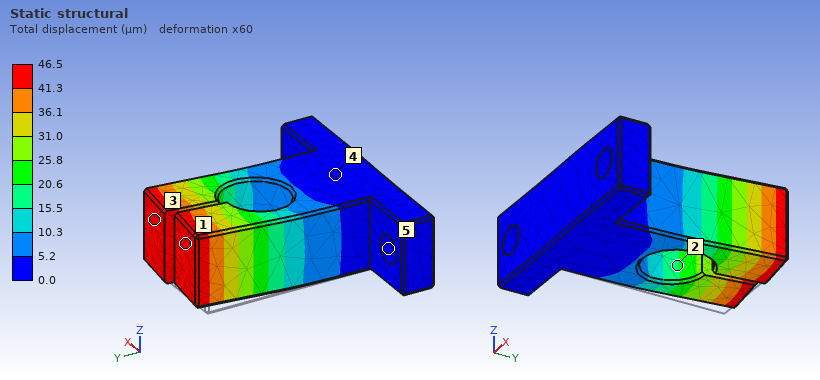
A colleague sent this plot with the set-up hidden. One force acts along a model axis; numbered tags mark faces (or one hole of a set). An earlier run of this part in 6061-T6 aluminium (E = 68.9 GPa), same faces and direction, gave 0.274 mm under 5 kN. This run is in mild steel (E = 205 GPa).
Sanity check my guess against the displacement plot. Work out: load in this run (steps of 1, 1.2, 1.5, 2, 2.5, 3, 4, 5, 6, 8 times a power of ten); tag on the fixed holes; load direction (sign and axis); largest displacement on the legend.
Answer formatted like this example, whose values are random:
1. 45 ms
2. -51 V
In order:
1. 2.5 kN
2. 5
3. +X
4. 46.5 µm
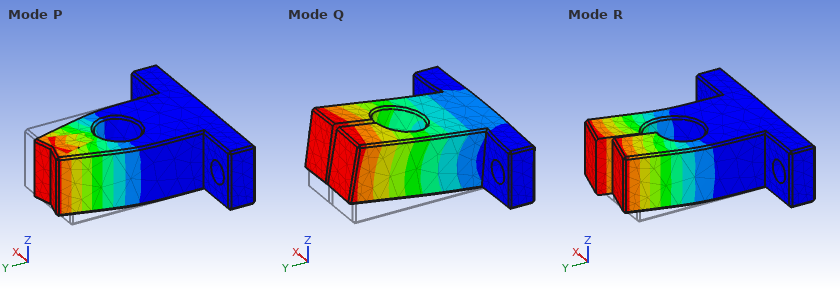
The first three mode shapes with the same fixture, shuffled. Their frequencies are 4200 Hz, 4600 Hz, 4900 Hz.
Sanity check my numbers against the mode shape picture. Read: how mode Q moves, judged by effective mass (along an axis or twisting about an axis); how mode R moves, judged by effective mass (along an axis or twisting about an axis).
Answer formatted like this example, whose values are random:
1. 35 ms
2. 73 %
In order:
1. along Z
2. along X
